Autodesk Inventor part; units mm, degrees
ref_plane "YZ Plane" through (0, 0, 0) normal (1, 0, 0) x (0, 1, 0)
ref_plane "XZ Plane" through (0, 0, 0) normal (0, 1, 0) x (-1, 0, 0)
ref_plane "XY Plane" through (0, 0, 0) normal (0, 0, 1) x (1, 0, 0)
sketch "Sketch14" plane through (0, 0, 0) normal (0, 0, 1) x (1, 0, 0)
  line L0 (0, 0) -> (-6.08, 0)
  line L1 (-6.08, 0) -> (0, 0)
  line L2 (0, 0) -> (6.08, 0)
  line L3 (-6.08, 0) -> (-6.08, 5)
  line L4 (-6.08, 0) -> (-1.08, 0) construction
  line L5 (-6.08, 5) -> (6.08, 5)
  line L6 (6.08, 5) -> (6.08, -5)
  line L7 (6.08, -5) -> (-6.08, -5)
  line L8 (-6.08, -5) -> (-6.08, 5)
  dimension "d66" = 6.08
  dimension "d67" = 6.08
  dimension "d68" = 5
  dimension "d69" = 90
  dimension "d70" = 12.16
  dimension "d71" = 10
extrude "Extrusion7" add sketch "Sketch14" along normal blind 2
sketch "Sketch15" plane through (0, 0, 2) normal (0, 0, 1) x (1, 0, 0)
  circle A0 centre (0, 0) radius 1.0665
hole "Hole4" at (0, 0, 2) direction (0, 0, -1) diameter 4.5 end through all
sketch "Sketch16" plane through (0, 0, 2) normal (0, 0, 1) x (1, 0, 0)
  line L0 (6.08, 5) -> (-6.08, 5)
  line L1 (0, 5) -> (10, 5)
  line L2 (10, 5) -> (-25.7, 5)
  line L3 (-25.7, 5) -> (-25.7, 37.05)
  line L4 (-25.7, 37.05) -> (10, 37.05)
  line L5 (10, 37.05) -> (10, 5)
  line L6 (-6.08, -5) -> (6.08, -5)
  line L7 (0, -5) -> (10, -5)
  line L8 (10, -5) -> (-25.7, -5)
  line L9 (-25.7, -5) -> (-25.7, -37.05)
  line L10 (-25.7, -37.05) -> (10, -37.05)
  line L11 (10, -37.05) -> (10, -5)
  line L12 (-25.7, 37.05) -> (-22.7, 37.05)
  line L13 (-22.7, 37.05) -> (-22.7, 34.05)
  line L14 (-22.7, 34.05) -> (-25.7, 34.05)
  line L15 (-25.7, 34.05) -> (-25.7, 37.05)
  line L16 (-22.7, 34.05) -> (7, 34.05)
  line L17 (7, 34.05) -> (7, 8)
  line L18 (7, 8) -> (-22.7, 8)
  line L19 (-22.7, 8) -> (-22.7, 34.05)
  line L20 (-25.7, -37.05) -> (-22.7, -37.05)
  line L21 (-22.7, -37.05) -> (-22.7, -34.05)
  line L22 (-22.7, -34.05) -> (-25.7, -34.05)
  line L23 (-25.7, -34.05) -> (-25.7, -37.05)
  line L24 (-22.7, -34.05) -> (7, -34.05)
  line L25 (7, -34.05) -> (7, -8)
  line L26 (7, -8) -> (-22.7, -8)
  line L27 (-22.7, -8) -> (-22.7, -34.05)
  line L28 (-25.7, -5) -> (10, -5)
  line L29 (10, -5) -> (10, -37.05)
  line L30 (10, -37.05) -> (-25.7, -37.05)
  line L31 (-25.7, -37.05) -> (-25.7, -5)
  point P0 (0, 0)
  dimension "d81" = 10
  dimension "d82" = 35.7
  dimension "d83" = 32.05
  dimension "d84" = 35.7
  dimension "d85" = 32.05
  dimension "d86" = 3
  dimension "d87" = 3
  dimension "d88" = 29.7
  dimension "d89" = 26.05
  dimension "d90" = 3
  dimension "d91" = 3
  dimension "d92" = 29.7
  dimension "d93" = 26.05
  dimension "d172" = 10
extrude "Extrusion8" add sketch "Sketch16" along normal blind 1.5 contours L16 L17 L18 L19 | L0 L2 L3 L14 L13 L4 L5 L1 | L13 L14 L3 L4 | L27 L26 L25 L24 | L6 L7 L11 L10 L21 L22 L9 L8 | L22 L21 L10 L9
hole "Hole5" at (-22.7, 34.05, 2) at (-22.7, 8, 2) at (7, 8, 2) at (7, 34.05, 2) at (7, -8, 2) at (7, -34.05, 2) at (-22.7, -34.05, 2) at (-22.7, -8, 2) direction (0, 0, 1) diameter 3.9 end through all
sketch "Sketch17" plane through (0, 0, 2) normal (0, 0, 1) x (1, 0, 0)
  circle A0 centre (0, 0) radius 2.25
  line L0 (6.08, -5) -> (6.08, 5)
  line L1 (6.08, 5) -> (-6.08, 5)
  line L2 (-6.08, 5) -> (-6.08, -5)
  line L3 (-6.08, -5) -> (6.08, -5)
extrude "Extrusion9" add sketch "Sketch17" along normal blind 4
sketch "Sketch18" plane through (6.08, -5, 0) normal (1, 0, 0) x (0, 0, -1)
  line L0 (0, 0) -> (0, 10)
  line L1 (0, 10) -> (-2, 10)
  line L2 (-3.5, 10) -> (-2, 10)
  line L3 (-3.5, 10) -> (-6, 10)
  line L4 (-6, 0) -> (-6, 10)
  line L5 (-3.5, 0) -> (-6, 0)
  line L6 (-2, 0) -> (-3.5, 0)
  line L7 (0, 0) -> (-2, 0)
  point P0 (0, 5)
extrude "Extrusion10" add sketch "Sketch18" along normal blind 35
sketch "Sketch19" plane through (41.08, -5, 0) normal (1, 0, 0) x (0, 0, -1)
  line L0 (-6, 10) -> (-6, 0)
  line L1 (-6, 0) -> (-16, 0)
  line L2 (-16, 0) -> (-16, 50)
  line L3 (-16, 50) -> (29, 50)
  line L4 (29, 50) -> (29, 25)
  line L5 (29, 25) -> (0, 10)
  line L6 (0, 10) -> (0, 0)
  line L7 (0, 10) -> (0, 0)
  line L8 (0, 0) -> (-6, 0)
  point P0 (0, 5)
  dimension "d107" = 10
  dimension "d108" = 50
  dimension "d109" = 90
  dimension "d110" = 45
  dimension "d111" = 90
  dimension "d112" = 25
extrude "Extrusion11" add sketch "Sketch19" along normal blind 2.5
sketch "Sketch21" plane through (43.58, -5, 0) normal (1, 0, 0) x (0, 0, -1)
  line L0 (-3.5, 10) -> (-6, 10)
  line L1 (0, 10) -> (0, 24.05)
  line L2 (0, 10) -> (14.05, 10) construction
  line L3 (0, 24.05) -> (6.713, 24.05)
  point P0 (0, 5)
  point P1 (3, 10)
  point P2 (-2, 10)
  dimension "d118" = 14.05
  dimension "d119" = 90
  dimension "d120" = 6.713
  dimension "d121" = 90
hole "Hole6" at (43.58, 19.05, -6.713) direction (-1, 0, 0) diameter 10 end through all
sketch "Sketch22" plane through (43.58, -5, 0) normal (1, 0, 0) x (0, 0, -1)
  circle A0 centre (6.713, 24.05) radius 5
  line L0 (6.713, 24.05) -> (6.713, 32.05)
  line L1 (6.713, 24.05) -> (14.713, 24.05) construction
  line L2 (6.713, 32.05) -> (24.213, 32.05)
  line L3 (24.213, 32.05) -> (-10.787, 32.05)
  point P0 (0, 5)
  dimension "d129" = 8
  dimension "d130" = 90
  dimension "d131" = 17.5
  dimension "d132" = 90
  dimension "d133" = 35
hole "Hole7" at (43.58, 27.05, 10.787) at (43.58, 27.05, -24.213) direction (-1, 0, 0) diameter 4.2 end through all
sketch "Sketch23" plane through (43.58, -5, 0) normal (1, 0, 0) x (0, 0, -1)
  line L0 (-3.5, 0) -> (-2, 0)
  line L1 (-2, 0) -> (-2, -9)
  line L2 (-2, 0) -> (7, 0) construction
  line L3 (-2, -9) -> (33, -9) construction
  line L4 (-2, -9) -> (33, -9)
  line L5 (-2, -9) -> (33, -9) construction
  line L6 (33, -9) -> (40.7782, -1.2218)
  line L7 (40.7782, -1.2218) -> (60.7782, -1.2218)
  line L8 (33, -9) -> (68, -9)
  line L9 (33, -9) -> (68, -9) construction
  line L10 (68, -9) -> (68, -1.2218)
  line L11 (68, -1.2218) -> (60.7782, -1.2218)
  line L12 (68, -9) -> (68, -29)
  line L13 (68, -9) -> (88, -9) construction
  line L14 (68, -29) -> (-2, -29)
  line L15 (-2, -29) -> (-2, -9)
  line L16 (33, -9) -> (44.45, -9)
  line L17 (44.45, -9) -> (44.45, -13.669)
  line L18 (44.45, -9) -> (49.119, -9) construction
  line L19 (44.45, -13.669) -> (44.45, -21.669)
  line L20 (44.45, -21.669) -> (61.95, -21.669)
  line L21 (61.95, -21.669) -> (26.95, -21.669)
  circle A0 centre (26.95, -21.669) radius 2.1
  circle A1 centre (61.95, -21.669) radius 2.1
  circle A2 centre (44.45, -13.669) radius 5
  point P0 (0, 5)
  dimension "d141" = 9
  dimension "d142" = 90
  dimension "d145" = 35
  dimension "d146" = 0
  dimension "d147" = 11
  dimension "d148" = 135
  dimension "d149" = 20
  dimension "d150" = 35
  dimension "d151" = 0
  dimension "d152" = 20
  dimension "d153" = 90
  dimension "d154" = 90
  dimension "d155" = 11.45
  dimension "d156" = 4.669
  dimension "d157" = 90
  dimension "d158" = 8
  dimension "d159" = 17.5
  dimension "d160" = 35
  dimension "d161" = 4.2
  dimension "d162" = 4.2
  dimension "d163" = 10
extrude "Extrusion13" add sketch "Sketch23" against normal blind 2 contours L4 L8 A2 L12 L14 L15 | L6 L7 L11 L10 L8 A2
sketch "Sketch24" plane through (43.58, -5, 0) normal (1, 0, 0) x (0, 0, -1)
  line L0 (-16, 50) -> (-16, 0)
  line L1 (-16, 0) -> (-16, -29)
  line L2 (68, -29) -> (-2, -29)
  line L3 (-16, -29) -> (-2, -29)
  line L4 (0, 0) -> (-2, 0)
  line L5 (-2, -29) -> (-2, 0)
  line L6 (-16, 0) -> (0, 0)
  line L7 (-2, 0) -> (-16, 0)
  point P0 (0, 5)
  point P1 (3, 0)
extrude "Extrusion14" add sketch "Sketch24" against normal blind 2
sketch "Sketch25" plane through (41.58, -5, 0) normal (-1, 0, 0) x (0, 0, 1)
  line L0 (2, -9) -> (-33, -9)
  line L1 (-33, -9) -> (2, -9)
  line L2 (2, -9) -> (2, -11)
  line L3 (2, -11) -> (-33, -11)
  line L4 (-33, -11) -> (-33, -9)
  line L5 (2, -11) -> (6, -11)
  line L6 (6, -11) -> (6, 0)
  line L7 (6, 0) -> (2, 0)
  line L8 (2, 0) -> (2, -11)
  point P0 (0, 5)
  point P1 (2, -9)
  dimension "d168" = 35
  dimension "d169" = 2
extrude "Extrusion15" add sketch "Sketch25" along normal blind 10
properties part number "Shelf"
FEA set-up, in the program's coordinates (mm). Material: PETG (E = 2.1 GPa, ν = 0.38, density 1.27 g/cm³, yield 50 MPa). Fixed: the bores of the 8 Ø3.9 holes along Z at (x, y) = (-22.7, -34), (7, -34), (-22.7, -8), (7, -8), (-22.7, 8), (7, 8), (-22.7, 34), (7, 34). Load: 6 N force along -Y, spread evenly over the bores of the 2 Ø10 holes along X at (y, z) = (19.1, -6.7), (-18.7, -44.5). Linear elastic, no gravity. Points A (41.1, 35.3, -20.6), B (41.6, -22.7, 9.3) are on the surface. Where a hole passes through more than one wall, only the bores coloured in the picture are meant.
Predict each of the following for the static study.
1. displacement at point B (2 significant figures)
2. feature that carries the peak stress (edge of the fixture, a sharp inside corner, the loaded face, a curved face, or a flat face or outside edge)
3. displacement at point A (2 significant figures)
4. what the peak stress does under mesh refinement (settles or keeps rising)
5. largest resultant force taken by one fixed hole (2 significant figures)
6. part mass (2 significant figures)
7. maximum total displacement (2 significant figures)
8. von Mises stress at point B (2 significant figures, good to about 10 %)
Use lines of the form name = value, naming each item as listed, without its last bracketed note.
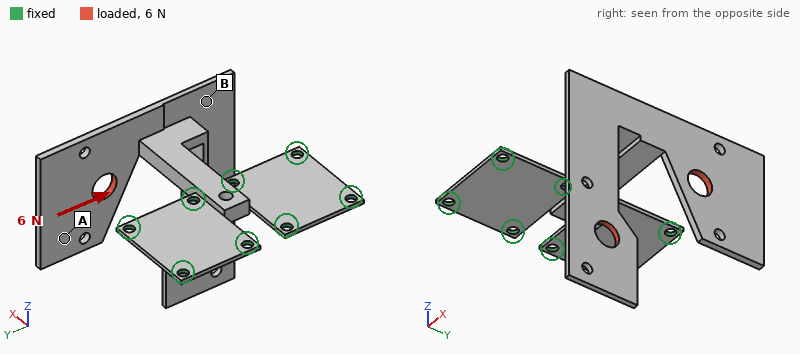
displacement at point B = 0.38 mm
feature that carries the peak stress = a sharp inside corner
displacement at point A = 0.73 mm
what the peak stress does under mesh refinement = keeps rising
largest resultant force taken by one fixed hole = 19 N
part mass = 19 g
maximum total displacement = 1.5 mm
von Mises stress at point B = 0.68 MPa
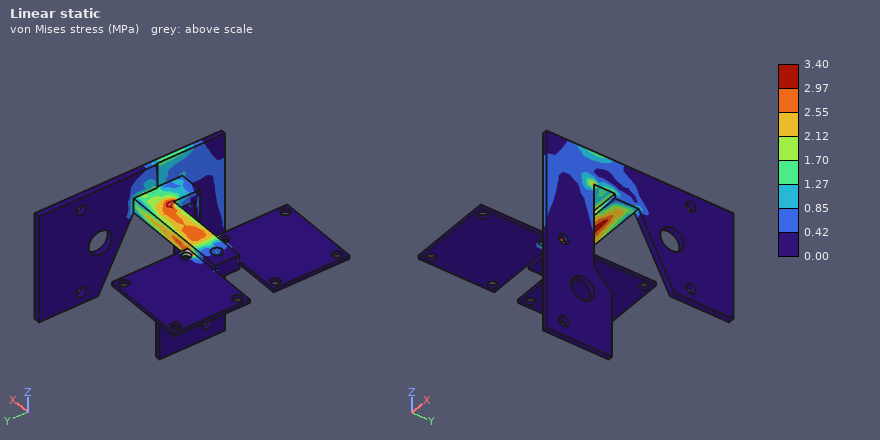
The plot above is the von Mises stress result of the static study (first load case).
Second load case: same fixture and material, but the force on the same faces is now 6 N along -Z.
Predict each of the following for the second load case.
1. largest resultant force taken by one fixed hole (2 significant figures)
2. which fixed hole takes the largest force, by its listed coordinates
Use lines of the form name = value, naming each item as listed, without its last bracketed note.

largest resultant force taken by one fixed hole = 5.9 N
which fixed hole takes the largest force, by its listed coordinates = (7, 8)
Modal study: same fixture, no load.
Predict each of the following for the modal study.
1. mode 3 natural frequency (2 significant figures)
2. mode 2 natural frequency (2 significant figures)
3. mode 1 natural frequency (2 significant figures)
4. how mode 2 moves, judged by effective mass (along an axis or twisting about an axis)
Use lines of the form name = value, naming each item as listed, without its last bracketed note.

mode 3 natural frequency = 160 Hz
mode 2 natural frequency = 120 Hz
mode 1 natural frequency = 97 Hz
how mode 2 moves, judged by effective mass = along Y
